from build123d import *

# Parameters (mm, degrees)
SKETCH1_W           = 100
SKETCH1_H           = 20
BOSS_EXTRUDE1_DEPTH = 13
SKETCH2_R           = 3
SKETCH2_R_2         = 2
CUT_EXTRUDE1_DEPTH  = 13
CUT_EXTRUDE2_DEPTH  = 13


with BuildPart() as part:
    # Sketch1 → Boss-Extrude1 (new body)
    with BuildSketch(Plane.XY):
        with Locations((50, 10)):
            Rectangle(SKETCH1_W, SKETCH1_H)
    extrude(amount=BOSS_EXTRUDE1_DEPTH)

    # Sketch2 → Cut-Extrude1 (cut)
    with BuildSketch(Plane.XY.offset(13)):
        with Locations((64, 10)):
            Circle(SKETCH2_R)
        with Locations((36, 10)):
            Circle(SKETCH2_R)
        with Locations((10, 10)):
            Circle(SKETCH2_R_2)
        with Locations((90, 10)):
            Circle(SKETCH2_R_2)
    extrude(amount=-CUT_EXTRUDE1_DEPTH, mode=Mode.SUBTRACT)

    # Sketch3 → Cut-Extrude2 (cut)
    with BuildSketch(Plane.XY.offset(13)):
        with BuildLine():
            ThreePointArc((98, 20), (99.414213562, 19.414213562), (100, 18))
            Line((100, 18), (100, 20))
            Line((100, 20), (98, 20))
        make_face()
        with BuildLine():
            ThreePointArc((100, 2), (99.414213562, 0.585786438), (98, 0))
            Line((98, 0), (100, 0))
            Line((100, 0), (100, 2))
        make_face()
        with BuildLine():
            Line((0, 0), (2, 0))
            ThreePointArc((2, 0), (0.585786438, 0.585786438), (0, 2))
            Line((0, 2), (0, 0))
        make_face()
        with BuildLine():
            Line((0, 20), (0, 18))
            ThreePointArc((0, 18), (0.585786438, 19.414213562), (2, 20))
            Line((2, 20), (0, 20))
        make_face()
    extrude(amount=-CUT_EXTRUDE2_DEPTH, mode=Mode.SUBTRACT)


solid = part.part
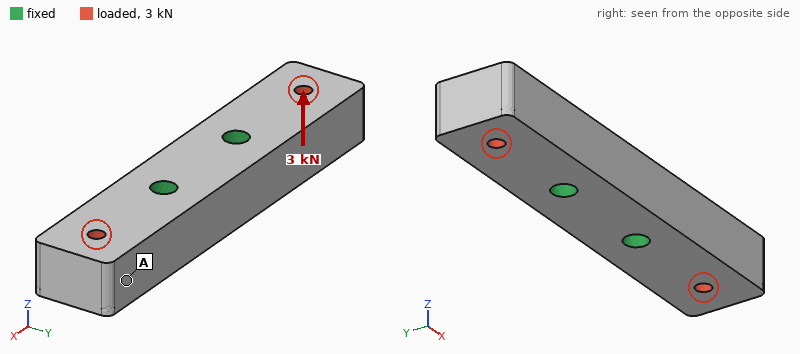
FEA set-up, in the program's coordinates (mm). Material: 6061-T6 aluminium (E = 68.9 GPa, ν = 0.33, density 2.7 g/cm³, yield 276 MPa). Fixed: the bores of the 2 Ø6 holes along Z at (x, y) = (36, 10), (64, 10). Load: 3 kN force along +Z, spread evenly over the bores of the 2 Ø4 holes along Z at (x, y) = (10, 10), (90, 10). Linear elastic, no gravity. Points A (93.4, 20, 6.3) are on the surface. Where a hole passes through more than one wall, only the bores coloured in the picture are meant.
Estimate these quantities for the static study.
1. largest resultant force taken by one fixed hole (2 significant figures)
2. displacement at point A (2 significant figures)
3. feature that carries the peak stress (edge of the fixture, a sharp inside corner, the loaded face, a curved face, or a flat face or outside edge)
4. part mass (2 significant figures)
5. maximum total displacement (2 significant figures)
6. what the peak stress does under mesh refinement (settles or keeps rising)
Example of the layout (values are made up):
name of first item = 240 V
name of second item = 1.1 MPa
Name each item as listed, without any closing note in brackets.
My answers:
largest resultant force taken by one fixed hole = 1.5 kN
displacement at point A = 47 µm
feature that carries the peak stress = edge of the fixture
part mass = 67 g
maximum total displacement = 62 µm
what the peak stress does under mesh refinement = keeps rising
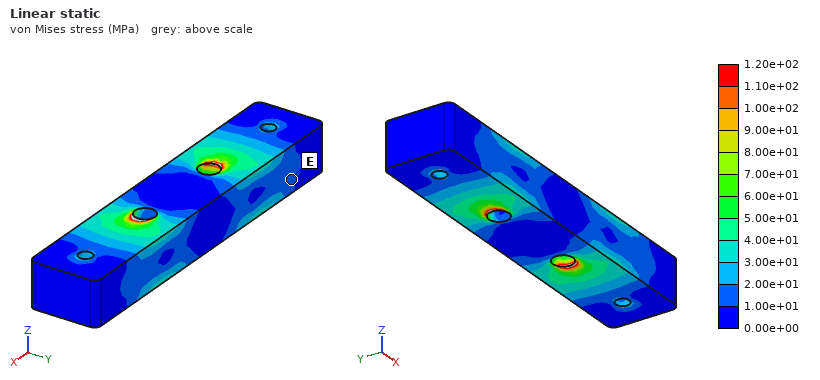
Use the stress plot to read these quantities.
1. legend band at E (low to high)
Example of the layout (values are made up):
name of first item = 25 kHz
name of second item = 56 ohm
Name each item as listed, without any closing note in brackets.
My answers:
legend band at E = 1.00e+01 to 2.00e+01 MPa
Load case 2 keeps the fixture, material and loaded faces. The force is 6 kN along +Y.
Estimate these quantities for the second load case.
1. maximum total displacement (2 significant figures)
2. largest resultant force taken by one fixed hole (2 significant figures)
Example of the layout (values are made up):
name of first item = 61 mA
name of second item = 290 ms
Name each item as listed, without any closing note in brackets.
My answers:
maximum total displacement = 91 µm
largest resultant force taken by one fixed hole = 3.0 kN
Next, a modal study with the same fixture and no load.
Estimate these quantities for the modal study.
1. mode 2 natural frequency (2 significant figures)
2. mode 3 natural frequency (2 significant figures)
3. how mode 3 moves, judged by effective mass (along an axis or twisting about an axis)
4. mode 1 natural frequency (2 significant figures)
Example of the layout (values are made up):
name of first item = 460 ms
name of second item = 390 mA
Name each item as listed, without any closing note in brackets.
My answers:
mode 2 natural frequency = 7700 Hz
mode 3 natural frequency = 8700 Hz
how mode 3 moves, judged by effective mass = along Y
mode 1 natural frequency = 7700 Hz
